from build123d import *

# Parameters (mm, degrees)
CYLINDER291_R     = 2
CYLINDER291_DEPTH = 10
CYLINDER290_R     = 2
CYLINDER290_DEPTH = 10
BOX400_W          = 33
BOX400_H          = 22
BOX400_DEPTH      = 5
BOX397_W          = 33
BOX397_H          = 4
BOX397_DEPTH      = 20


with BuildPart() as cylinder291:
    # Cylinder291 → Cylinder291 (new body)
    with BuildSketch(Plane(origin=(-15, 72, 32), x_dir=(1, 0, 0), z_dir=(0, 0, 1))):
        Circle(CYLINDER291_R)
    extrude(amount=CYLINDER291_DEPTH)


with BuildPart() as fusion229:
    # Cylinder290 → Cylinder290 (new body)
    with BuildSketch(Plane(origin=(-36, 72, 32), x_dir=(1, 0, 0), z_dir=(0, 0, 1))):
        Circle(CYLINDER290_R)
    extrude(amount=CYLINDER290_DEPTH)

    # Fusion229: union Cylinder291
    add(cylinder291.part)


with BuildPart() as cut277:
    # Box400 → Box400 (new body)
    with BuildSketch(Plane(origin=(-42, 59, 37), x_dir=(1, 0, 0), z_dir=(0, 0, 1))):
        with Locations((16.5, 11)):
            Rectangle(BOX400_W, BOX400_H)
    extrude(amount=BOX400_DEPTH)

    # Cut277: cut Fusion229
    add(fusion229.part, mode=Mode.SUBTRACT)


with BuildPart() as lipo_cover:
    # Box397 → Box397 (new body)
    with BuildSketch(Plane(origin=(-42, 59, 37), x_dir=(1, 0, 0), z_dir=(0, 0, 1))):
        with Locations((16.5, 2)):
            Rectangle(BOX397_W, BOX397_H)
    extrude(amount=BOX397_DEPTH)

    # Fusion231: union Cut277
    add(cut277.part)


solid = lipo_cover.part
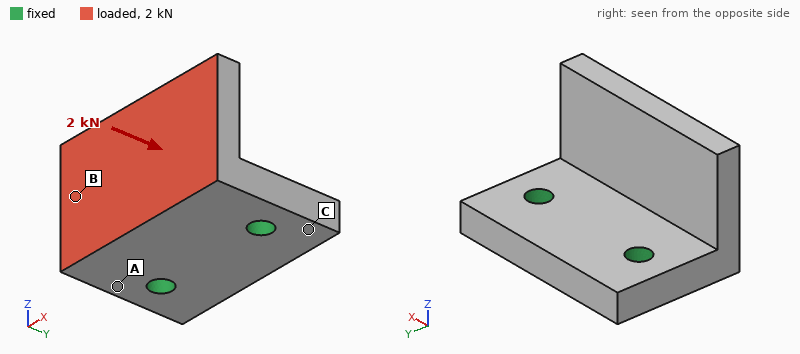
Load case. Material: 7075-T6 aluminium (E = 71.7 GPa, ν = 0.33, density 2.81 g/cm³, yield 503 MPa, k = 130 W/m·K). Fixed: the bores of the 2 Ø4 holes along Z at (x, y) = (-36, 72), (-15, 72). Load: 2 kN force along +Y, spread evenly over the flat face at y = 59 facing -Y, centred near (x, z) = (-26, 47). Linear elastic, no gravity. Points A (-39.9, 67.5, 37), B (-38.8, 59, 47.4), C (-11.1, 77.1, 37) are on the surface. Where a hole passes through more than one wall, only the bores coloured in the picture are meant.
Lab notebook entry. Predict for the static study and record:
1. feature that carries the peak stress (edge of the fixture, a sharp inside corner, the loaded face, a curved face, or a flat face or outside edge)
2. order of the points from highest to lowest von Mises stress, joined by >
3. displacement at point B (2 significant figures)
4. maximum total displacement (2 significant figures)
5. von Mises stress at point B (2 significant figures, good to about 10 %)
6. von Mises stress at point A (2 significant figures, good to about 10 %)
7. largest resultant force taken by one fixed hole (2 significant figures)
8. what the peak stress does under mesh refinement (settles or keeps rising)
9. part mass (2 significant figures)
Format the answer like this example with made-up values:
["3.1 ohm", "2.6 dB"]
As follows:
["edge of the fixture", "A > B > C", "0.089 mm", "0.19 mm", "53 MPa", "96 MPa", "1.0 kN", "keeps rising", "15 g"]
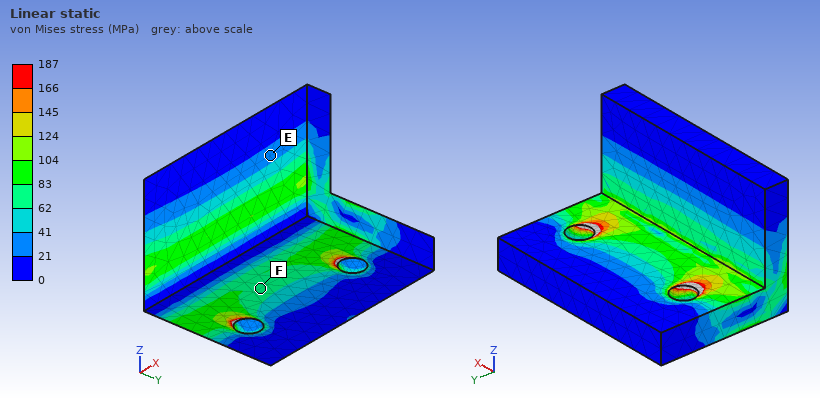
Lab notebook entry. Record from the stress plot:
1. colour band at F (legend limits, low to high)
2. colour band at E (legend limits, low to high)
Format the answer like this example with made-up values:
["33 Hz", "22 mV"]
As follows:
["62 to 83 MPa", "21 to 41 MPa"]
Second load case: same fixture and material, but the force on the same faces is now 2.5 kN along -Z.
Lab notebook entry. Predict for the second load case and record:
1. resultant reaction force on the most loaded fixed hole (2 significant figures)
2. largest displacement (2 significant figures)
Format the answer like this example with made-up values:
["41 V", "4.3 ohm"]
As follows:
["1.3 kN", "0.19 mm"]
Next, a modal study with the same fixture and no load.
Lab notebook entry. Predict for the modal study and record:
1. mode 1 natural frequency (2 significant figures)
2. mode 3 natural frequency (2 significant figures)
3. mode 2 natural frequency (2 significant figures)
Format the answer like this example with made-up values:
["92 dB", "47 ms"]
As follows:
["6900 Hz", "17 kHz", "12 kHz"]
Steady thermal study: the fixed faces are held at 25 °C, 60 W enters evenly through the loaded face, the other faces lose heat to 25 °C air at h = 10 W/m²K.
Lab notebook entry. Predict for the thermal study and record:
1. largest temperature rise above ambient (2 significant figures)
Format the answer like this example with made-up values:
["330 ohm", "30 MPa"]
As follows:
["54 K"]
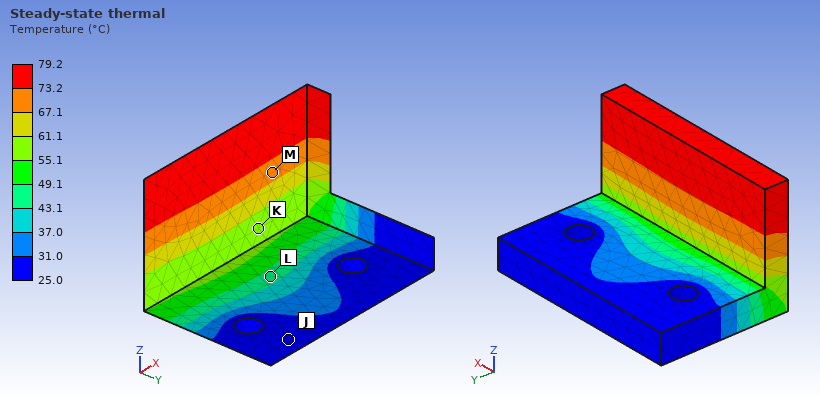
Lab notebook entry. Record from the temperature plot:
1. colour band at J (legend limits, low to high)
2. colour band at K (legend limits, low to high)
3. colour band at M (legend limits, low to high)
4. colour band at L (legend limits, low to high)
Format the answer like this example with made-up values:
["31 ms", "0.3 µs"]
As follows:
["25.0 to 31.0 °C", "55.1 to 61.1 °C", "67.1 to 73.2 °C", "43.1 to 49.1 °C"]
